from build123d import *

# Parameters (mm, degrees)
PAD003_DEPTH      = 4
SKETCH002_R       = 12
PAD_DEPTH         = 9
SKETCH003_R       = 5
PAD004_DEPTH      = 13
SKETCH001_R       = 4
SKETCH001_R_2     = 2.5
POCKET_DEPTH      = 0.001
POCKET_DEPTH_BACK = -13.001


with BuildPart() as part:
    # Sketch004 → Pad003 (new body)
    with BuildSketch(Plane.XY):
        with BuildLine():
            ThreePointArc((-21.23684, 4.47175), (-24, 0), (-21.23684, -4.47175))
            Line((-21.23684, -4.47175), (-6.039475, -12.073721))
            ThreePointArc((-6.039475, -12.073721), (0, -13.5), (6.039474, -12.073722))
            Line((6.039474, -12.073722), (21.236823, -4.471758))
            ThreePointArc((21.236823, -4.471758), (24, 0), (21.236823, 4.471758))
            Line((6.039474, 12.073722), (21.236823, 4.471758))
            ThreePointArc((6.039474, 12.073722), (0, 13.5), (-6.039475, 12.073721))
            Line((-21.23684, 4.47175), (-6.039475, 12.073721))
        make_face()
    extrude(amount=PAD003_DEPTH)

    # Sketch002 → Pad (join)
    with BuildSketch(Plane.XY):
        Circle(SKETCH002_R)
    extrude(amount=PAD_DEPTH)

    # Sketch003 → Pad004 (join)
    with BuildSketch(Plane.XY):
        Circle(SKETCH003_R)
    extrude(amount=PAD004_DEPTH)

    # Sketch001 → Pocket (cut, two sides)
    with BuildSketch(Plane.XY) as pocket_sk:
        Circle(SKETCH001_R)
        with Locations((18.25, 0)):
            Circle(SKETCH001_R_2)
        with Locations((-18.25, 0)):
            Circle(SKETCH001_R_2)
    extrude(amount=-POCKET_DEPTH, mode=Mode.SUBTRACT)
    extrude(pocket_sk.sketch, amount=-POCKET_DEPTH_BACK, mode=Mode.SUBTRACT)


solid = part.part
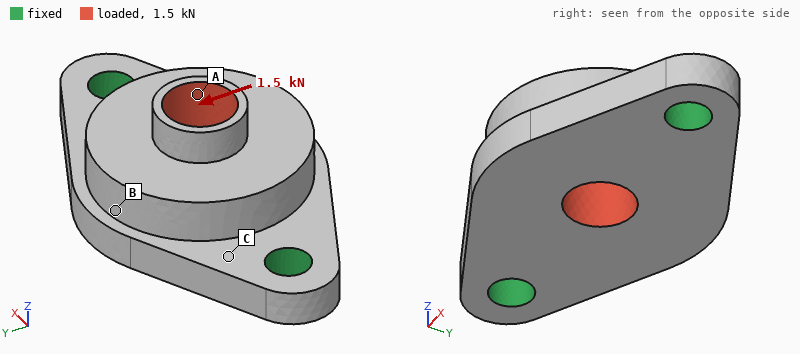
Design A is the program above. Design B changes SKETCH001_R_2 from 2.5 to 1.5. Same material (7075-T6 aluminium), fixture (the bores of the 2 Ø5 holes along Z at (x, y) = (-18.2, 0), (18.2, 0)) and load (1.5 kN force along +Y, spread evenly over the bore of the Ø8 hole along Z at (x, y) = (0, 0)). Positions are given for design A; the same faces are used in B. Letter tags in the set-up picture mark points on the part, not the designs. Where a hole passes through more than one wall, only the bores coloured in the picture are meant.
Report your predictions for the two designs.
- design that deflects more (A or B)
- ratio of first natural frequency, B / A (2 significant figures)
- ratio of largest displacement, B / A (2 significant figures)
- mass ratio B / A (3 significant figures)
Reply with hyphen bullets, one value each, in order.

- B
- 0.84
- 1.3
- 1.02
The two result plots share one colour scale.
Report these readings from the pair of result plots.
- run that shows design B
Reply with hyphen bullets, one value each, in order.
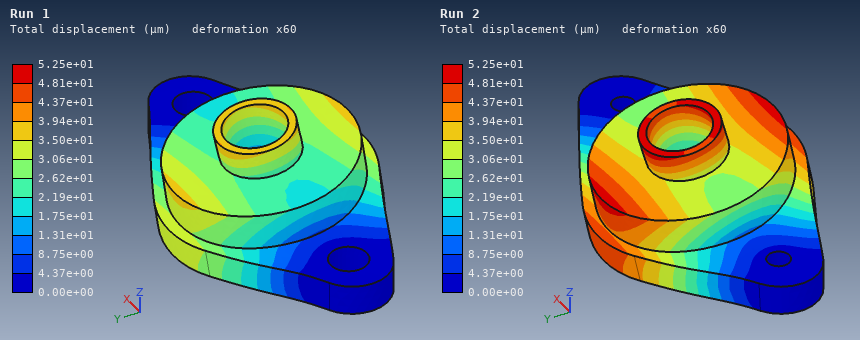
- Run 2
